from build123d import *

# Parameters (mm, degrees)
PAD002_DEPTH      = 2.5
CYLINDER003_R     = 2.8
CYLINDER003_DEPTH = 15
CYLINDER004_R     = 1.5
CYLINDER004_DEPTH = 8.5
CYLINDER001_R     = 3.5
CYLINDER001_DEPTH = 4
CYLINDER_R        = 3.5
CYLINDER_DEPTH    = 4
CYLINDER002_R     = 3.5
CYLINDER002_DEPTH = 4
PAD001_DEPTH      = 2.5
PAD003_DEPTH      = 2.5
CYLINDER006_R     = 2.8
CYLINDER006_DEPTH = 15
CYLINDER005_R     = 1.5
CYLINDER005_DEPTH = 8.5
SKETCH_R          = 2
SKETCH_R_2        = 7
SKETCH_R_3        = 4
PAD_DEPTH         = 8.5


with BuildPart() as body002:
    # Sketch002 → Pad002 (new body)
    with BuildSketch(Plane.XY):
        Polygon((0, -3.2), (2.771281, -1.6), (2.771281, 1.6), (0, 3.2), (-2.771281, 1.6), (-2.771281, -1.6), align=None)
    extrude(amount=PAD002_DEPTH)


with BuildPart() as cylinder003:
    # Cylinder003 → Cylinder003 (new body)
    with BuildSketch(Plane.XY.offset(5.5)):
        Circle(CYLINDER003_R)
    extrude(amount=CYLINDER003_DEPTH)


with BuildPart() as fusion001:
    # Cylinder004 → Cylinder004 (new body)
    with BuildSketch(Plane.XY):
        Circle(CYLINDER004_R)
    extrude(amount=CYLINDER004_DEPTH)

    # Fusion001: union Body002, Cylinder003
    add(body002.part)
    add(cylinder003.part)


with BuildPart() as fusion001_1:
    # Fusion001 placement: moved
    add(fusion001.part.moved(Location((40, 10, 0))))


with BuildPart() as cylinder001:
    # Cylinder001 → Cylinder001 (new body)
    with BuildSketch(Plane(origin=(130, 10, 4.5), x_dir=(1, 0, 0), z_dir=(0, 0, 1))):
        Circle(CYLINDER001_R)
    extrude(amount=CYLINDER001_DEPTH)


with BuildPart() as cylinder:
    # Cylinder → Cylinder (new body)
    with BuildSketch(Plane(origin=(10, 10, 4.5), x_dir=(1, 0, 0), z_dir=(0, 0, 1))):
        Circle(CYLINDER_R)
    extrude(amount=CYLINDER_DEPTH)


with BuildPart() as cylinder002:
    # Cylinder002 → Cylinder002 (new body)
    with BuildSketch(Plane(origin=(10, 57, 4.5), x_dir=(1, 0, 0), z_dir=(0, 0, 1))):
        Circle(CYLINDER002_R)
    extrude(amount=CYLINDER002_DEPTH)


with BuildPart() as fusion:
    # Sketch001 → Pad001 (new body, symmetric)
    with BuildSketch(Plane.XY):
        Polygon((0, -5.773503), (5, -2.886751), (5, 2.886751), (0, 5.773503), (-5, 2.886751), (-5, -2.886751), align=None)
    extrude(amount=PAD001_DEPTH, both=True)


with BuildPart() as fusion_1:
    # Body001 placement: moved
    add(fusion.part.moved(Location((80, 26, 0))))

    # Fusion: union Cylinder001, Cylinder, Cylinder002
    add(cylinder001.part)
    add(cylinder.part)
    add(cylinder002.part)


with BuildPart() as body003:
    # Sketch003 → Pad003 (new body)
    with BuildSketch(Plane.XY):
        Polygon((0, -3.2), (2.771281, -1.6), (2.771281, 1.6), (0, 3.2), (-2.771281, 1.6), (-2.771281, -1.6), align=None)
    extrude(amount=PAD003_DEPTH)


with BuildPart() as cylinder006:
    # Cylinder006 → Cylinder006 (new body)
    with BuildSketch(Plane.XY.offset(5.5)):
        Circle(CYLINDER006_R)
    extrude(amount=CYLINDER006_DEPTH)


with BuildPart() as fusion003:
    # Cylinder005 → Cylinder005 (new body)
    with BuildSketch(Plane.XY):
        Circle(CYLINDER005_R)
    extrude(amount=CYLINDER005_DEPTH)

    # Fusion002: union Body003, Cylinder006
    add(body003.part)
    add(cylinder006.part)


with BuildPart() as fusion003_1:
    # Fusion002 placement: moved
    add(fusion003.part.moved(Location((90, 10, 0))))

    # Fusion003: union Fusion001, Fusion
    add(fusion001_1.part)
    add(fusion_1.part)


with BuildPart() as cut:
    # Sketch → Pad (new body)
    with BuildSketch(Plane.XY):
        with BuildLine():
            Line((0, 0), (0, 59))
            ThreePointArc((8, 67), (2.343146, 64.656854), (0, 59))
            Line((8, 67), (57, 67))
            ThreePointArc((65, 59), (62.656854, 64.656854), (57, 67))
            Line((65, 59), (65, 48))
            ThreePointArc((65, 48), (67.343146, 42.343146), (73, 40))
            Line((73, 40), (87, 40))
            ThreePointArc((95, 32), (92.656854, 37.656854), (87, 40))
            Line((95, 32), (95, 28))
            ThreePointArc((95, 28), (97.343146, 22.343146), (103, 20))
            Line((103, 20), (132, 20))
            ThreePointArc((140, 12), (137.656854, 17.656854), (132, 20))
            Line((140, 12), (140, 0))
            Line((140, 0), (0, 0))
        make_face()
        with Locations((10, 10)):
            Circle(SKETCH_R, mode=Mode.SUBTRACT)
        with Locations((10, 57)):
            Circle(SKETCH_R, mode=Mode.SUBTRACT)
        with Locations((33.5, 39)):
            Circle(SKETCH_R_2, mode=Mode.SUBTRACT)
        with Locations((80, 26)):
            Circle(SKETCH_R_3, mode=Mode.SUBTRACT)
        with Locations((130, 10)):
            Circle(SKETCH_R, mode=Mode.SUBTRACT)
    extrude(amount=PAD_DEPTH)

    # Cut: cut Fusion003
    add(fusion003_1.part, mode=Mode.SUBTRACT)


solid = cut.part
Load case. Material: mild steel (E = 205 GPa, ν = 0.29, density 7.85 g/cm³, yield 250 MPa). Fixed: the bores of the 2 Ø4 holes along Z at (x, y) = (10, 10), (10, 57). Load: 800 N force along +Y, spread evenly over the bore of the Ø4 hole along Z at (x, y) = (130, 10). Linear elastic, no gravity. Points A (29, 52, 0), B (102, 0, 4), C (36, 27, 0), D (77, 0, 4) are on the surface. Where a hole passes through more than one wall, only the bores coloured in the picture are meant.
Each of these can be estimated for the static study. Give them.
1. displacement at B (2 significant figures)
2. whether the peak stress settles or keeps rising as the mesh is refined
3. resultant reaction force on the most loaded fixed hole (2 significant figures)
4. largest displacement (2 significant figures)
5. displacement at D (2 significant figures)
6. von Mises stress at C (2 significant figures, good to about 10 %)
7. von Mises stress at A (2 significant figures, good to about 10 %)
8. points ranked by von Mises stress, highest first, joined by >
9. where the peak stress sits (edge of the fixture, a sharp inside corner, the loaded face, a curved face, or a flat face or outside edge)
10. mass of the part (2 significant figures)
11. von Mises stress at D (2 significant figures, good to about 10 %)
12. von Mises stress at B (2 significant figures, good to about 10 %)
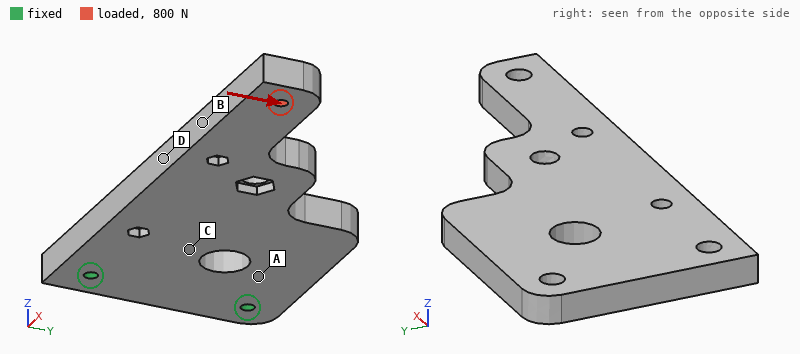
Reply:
26 µm
keeps rising
2.0 kN
61 µm
15 µm
8.7 MPa
17 MPa
B > D > A > C
edge of the fixture
410 g
27 MPa
38 MPa
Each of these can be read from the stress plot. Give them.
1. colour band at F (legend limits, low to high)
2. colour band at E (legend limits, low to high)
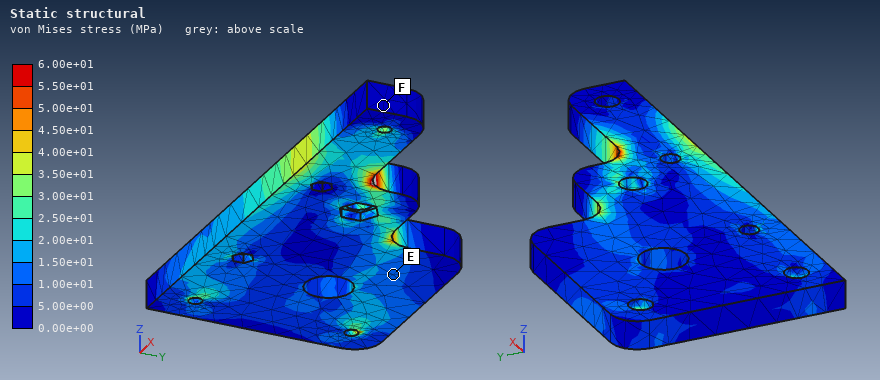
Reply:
0.00e+00 to 5.00e+00 MPa
1.00e+01 to 1.50e+01 MPa
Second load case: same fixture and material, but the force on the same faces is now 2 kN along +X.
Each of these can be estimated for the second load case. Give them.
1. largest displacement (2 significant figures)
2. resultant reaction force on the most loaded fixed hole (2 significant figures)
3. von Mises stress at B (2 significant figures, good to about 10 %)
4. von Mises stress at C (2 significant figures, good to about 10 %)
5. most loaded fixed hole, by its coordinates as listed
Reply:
83 µm
2.0 kN
14 MPa
11 MPa
(10, 10)
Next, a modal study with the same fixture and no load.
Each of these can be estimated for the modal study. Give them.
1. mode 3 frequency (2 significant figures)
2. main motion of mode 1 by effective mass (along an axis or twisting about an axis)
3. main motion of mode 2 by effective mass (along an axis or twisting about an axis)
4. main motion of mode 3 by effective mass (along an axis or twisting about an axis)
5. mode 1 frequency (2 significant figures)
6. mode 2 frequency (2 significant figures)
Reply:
3000 Hz
along Z
along Z
along Y
490 Hz
2100 Hz
